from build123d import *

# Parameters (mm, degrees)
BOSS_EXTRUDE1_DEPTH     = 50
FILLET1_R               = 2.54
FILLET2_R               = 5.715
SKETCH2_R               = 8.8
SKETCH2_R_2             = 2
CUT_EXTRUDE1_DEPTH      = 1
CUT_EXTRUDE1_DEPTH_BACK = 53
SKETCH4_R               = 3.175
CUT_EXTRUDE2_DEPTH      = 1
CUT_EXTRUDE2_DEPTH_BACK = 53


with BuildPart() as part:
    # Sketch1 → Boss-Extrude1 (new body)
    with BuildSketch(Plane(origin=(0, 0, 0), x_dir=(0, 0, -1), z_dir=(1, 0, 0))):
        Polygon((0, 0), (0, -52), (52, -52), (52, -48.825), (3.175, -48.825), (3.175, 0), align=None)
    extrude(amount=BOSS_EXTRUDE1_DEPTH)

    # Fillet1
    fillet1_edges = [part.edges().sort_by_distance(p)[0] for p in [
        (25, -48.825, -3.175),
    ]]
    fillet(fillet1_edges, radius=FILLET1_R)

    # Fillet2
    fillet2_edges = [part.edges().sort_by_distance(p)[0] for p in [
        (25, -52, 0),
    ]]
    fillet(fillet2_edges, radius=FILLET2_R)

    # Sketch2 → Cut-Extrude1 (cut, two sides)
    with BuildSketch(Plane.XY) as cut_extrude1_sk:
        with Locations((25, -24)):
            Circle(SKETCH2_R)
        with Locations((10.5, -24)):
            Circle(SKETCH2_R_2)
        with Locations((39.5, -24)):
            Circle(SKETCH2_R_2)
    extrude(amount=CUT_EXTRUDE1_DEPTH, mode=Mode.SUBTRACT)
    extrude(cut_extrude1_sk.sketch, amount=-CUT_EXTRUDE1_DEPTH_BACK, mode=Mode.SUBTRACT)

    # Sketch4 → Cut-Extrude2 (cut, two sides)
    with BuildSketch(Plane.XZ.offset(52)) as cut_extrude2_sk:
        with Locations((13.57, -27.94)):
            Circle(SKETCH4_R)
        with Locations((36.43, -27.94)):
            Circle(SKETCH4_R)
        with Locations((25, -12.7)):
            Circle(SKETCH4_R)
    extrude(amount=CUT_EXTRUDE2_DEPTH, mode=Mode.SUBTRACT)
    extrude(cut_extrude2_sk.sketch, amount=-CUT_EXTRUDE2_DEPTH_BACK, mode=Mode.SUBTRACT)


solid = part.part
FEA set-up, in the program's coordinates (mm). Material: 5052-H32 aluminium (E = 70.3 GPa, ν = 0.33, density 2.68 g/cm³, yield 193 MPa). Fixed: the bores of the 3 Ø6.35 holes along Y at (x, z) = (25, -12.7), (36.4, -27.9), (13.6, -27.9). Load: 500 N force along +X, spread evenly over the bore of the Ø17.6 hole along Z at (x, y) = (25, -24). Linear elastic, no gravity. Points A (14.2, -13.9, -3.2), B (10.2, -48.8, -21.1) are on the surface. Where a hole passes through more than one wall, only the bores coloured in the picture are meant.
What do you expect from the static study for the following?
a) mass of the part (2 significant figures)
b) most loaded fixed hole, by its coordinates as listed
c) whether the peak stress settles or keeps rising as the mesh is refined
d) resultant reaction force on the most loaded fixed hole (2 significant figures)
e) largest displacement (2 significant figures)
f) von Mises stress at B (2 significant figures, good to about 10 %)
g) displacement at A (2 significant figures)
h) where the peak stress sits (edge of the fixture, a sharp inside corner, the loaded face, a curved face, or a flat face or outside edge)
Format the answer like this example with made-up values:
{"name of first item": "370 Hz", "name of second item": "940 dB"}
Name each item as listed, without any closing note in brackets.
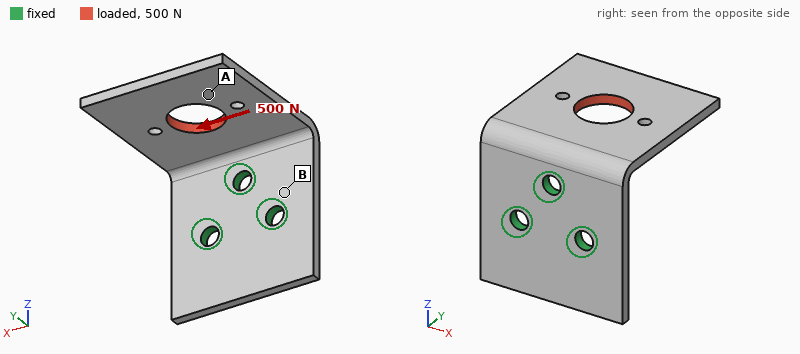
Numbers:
{"mass of the part": "39 g", "most loaded fixed hole, by its coordinates as listed": "(25, -12.7)", "whether the peak stress settles or keeps rising as the mesh is refined": "keeps rising", "resultant reaction force on the most loaded fixed hole": "480 N", "largest displacement": "0.43 mm", "von Mises stress at B": "59 MPa", "displacement at A": "0.29 mm", "where the peak stress sits": "edge of the fixture"}
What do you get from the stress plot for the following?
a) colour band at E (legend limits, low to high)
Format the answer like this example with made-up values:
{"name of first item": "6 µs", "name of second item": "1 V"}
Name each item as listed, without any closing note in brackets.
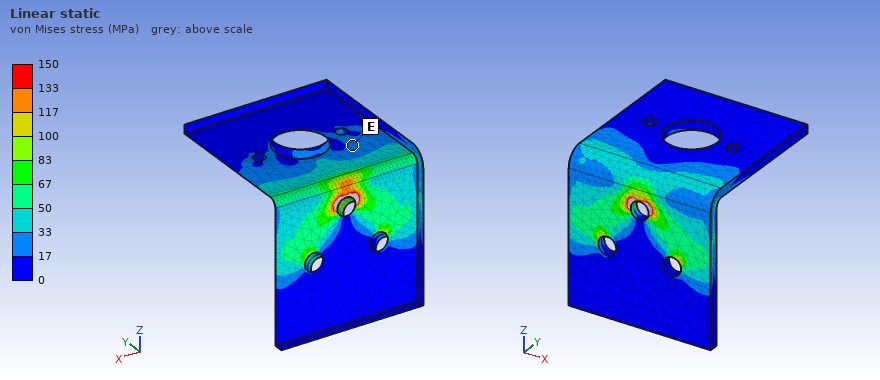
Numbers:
{"colour band at E": "17 to 33 MPa"}
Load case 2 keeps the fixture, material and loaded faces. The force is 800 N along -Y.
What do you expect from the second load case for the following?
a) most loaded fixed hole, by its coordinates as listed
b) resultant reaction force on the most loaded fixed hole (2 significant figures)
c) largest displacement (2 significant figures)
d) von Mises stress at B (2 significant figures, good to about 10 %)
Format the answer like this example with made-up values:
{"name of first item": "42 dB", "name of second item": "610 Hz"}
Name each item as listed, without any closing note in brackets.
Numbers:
{"most loaded fixed hole, by its coordinates as listed": "(25, -12.7)", "resultant reaction force on the most loaded fixed hole": "940 N", "largest displacement": "0.27 mm", "von Mises stress at B": "15 MPa"}
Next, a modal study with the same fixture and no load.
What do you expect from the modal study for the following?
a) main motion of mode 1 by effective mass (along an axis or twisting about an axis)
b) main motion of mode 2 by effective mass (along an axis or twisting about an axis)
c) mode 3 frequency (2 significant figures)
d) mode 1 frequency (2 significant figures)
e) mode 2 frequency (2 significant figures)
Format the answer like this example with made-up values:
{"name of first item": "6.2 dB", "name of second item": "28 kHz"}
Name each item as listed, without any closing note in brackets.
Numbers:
{"main motion of mode 1 by effective mass": "along Z", "main motion of mode 2 by effective mass": "along X", "mode 3 frequency": "2300 Hz", "mode 1 frequency": "800 Hz", "mode 2 frequency": "1400 Hz"}
